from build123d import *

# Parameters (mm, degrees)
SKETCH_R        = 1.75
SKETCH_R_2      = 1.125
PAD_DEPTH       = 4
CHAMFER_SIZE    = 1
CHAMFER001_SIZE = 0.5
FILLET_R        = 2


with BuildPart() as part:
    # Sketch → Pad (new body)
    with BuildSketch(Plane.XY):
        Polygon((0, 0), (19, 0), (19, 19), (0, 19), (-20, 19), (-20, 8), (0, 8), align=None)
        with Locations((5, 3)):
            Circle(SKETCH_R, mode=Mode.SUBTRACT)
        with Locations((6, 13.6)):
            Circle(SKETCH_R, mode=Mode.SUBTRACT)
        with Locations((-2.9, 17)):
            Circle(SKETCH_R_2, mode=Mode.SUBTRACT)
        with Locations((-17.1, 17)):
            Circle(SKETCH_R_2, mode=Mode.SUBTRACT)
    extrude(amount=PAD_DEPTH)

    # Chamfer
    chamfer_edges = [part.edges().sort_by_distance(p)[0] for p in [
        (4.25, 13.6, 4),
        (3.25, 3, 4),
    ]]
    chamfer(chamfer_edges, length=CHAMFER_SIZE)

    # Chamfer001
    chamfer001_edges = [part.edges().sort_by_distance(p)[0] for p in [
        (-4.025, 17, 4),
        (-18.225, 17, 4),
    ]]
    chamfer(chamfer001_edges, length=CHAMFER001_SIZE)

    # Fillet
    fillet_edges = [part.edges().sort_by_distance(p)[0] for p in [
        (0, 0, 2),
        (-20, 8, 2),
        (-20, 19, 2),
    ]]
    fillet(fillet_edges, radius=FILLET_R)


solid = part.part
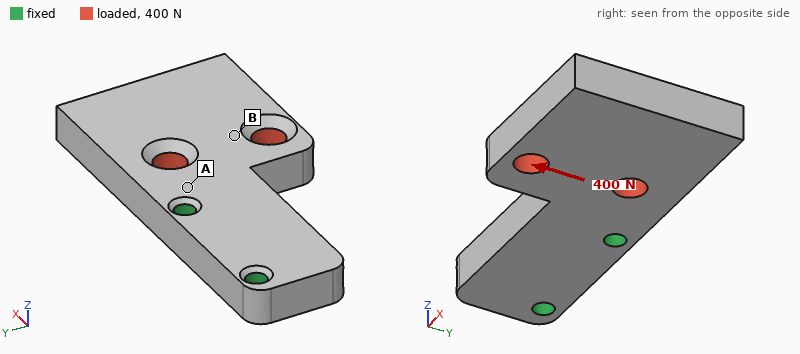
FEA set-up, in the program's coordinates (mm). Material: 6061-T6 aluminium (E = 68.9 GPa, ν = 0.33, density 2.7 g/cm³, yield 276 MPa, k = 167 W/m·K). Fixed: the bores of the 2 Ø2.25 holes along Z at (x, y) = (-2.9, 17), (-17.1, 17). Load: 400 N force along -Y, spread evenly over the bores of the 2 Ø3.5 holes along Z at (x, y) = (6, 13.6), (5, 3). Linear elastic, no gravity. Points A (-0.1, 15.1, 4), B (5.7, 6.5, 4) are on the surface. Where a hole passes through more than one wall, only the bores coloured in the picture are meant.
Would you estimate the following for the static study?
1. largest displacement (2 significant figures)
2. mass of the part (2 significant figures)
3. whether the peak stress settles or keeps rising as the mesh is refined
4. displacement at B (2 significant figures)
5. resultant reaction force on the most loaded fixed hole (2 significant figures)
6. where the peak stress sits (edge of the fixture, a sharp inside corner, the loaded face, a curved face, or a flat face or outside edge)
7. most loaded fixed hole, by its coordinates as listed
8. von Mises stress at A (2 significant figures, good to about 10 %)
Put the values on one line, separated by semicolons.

30 µm; 5.9 g; keeps rising; 13 µm; 610 N; edge of the fixture; (-2.9, 17); 20 MPa
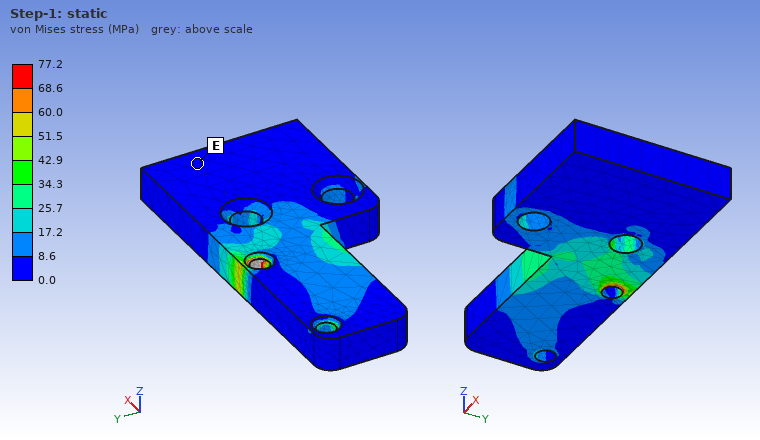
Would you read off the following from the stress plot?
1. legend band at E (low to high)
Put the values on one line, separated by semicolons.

0.0 to 8.6 MPa
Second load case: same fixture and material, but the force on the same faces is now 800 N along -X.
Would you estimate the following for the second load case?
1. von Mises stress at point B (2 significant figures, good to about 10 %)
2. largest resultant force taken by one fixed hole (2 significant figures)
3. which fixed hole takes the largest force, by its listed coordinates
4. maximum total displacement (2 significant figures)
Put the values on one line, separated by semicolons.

14 MPa; 620 N; (-17.1, 17); 59 µm
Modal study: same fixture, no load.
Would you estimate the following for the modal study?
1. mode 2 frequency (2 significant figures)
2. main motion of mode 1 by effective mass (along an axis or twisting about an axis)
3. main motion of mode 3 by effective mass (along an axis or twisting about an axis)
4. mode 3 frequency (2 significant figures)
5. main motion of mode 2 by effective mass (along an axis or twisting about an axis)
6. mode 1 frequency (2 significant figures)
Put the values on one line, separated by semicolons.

8800 Hz; along Z; twisting about X; 9500 Hz; along Y; 4100 Hz
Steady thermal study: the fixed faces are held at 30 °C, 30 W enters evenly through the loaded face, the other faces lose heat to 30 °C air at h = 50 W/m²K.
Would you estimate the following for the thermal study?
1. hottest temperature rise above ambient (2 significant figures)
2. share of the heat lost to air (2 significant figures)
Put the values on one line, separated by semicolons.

54 K; 6.8 %
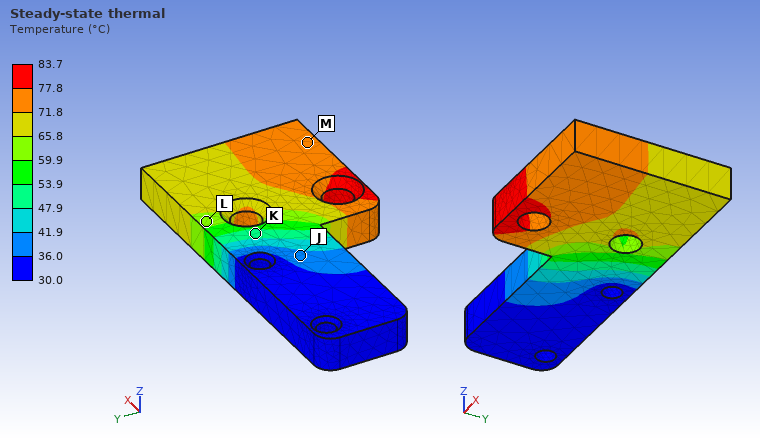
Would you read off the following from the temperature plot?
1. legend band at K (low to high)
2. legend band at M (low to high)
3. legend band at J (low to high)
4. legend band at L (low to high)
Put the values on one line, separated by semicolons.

47.9 to 53.9 °C; 71.8 to 77.8 °C; 36.0 to 41.9 °C; 59.9 to 65.8 °C
